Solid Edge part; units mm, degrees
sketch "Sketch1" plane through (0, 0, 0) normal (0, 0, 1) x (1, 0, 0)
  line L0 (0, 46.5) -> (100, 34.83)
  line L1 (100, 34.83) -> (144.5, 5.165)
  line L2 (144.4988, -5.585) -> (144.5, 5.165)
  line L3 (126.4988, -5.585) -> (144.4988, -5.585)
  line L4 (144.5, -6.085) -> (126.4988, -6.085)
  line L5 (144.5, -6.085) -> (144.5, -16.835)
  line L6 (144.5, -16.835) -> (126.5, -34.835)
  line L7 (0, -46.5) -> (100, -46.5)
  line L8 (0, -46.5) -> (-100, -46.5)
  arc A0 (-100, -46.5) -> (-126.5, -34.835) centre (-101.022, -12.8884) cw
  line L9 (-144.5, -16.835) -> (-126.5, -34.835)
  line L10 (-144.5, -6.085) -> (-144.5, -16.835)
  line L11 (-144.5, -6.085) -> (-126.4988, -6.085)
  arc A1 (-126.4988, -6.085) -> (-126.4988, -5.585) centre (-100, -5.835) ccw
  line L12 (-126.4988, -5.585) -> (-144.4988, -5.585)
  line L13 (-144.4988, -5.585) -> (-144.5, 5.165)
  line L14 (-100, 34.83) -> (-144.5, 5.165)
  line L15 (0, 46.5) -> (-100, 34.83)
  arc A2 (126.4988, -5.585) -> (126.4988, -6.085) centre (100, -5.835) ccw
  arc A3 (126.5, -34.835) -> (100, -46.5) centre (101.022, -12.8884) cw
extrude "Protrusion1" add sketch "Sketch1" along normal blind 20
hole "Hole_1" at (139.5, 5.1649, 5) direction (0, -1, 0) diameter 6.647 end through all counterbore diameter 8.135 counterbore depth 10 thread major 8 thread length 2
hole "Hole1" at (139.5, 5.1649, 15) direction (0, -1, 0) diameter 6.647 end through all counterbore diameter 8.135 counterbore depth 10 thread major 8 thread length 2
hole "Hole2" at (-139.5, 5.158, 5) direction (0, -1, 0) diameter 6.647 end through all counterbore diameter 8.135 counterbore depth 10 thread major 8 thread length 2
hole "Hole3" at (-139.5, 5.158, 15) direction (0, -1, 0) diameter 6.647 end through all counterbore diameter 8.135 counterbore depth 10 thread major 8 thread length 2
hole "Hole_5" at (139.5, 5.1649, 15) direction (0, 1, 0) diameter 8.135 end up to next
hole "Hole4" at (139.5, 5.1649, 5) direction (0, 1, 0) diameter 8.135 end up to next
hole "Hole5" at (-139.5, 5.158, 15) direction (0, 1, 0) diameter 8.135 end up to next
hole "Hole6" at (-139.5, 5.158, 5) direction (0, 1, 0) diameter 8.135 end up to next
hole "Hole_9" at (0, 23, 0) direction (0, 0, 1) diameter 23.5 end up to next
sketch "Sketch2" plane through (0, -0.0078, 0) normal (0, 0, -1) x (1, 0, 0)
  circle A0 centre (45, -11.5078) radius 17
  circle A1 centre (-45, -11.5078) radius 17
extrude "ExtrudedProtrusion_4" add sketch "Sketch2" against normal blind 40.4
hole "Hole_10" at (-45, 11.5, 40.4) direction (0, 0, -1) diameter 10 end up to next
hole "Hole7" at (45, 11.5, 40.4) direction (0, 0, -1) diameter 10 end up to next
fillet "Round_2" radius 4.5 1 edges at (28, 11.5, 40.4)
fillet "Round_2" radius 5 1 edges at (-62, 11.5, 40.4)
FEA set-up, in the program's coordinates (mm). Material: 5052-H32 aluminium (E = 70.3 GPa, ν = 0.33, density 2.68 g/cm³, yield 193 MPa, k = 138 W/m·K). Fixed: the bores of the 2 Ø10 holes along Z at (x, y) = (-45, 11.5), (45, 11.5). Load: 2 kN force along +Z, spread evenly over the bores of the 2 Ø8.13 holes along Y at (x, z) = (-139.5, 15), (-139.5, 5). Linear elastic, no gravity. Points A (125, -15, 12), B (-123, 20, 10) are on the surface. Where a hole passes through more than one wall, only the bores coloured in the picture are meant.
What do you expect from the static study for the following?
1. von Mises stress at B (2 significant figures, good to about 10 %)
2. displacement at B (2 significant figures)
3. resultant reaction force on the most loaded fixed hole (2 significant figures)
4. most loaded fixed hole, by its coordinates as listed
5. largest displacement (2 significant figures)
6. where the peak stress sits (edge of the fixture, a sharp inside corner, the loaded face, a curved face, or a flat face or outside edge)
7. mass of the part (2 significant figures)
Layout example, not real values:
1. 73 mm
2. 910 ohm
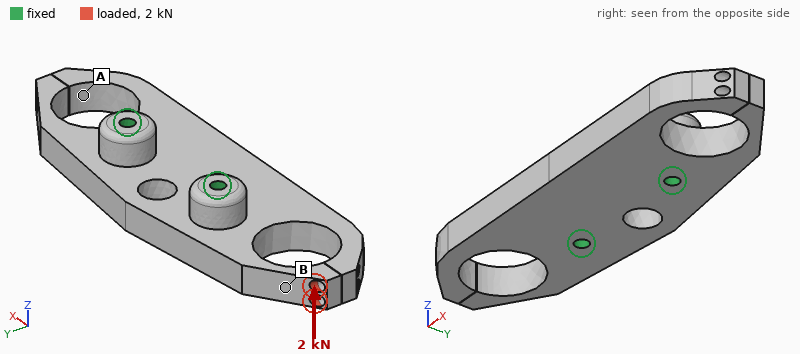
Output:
1. 59 MPa
2. 0.32 mm
3. 2.4 kN
4. (-45, 11.5)
5. 0.65 mm
6. a curved face
7. 1.0 kg
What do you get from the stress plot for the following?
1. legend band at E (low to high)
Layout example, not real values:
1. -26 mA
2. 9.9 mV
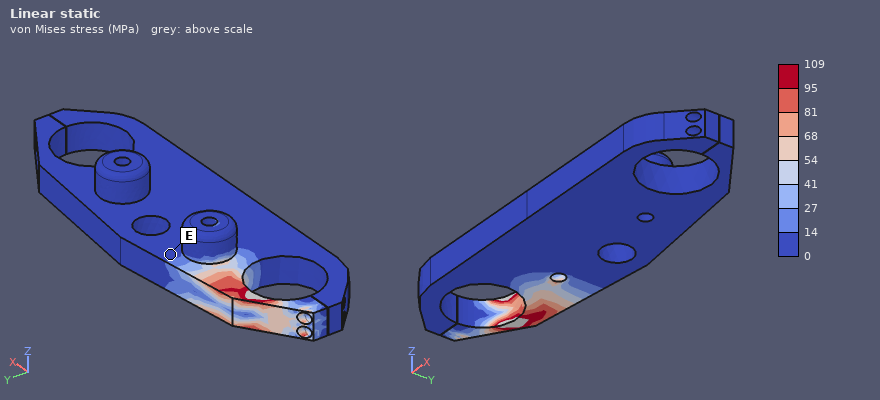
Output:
1. 0 to 14 MPa
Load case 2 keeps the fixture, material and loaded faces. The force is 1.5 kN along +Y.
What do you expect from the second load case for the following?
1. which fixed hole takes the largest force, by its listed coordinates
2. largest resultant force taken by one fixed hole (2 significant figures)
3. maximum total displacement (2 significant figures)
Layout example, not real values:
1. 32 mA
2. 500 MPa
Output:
1. (-45, 11.5)
2. 2.7 kN
3. 0.84 mm
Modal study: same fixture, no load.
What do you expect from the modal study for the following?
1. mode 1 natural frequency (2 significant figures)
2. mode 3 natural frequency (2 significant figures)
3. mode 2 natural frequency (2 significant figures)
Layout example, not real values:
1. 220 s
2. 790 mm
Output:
1. 1800 Hz
2. 2100 Hz
3. 1800 Hz
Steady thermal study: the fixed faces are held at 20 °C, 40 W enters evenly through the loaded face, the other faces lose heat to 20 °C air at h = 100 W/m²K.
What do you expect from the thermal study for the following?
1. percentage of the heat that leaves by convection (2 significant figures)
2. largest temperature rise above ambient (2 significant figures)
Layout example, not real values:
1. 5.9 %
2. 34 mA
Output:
1. 54 %
2. 67 K
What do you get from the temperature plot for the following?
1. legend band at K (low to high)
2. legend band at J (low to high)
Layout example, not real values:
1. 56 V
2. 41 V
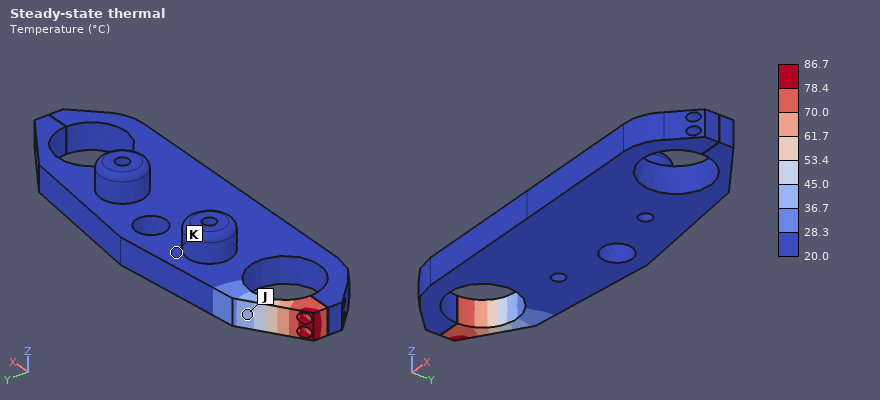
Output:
1. 20.0 to 28.3 °C
2. 36.7 to 45.0 °C
